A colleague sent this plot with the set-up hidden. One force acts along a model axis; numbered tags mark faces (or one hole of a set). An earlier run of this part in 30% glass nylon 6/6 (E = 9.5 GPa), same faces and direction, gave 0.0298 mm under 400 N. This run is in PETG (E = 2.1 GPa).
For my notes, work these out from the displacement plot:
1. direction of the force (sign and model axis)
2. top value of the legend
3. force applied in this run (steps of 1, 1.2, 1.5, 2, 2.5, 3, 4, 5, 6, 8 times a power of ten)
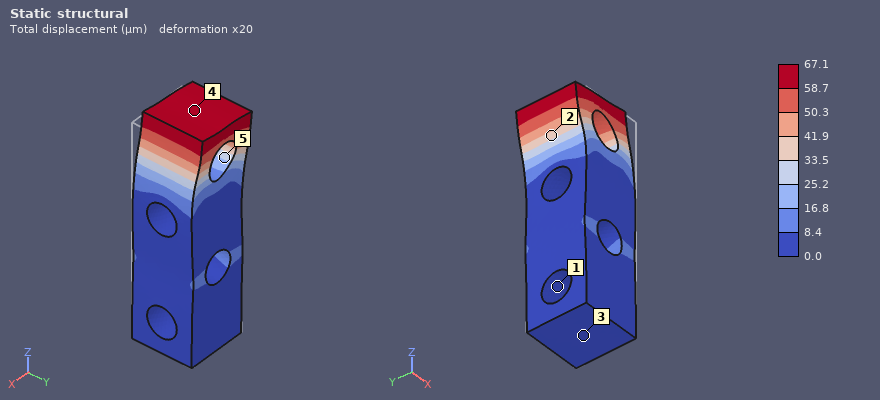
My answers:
-X
67.1 µm
200 N
